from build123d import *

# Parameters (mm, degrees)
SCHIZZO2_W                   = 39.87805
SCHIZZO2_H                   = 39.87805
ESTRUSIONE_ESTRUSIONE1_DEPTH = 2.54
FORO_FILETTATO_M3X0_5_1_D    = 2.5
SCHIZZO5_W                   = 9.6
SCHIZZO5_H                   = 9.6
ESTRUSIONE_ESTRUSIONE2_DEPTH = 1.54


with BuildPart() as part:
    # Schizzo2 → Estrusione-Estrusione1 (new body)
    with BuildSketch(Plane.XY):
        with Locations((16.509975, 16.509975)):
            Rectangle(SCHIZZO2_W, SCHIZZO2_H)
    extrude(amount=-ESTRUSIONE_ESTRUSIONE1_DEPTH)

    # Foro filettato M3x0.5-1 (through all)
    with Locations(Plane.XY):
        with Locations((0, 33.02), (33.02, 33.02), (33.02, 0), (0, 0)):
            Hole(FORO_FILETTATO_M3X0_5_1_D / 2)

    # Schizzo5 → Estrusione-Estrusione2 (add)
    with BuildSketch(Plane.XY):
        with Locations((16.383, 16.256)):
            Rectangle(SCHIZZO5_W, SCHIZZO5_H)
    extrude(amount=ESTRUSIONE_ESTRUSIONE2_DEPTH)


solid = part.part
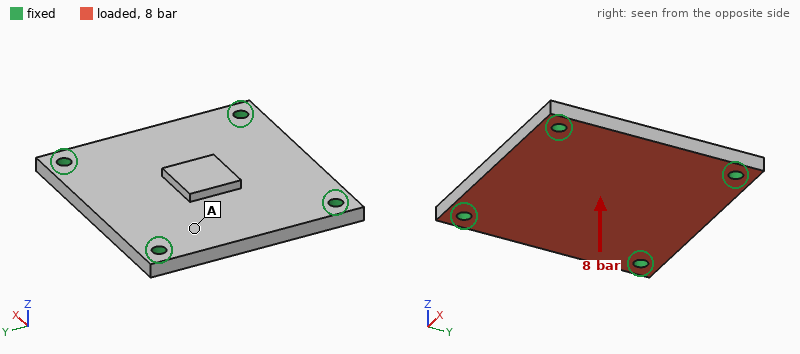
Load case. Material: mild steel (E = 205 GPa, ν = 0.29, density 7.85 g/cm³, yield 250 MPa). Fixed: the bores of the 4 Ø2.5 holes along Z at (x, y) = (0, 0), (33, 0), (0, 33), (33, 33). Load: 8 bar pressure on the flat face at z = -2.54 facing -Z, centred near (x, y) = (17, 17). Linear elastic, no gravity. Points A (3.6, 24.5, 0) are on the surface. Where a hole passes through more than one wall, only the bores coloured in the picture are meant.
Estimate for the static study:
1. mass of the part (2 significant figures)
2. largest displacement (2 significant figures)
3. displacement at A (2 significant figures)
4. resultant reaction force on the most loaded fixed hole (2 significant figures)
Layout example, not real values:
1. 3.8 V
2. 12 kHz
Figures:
1. 32 g
2. 20 µm
3. 11 µm
4. 310 N
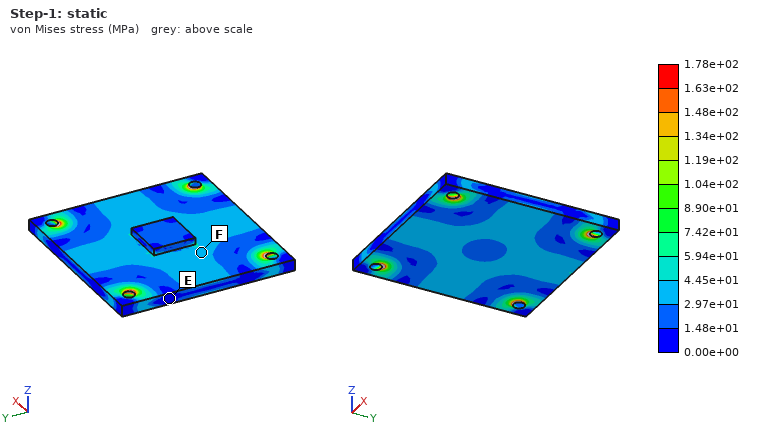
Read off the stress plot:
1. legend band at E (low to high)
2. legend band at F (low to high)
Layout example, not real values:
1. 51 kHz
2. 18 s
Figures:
1. 0.00e+00 to 1.48e+01 MPa
2. 2.97e+01 to 4.45e+01 MPa
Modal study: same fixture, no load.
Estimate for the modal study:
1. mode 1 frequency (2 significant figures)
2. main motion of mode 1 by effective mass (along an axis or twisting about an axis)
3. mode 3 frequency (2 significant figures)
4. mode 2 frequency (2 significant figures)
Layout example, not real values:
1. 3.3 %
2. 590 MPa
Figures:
1. 7900 Hz
2. along Z
3. 13 kHz
4. 13 kHz
